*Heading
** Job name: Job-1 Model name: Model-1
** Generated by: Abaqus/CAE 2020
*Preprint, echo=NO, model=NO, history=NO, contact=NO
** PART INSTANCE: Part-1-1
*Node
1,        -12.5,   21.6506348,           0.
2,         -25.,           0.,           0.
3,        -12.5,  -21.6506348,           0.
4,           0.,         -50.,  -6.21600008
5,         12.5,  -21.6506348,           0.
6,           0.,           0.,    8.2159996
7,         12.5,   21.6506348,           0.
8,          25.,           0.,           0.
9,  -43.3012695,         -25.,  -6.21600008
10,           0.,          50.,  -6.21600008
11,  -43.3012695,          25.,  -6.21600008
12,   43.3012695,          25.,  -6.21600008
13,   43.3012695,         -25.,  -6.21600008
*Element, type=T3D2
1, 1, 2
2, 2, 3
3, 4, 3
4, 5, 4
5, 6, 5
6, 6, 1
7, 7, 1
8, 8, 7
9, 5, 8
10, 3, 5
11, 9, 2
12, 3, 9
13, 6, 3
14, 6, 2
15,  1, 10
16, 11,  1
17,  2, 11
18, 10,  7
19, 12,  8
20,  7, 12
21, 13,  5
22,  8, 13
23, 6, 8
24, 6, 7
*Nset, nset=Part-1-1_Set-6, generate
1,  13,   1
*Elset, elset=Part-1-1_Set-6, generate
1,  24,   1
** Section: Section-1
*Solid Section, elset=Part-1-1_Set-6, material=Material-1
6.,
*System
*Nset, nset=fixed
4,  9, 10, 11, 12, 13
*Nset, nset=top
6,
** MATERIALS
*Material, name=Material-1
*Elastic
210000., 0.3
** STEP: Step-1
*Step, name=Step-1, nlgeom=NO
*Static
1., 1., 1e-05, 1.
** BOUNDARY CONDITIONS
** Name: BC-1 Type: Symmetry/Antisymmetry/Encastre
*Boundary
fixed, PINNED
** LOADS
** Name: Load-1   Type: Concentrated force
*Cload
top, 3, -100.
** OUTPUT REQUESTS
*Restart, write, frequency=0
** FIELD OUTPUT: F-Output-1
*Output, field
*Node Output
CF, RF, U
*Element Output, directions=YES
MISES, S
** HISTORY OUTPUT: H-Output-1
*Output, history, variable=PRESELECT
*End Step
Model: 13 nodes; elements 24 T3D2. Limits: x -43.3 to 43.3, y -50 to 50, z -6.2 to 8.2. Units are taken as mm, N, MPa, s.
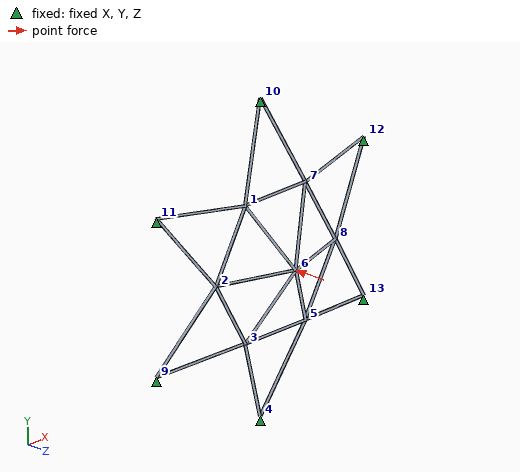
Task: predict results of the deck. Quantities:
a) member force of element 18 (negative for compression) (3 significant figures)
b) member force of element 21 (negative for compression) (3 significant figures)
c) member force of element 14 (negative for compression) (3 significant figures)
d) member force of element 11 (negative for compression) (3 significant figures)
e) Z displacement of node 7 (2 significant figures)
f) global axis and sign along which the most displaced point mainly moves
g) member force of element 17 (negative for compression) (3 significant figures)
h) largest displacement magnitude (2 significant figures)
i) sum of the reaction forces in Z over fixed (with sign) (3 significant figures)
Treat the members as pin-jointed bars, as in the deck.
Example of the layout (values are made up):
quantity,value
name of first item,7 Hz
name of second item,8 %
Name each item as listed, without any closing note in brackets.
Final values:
quantity,value
member force of element 18 (negative for compression),-42.4 N
member force of element 21 (negative for compression),-42.4 N
member force of element 14 (negative for compression),-53.4 N
member force of element 11 (negative for compression),-42.4 N
Z displacement of node 7,-0.0053 mm
global axis and sign along which the most displaced point mainly moves,-Z
member force of element 17 (negative for compression),-42.4 N
largest displacement magnitude,0.0090 mm
sum of the reaction forces in Z over fixed (with sign),100 N
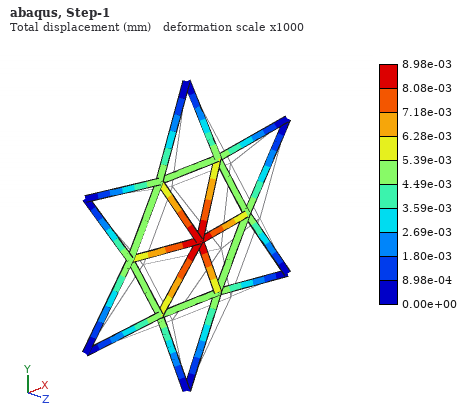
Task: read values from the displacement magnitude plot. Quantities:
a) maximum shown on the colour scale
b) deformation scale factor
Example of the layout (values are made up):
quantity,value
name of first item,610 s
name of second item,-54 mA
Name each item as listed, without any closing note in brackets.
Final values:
quantity,value
maximum shown on the colour scale,8.98e-03 mm
deformation scale factor,1000
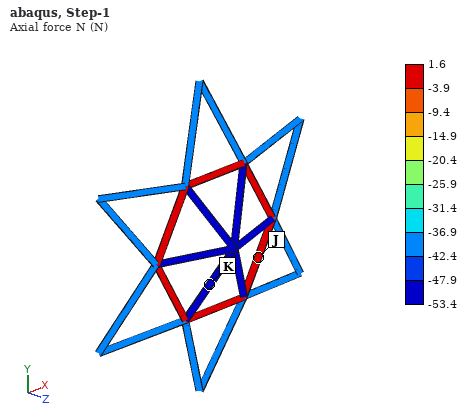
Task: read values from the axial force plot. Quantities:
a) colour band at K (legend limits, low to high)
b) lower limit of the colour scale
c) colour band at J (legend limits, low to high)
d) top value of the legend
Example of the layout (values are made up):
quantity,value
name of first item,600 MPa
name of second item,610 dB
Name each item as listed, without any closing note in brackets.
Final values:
quantity,value
colour band at K,-53.4 to -47.9 N
lower limit of the colour scale,-53.4 N
colour band at J,-3.9 to 1.6 N
top value of the legend,1.6 N
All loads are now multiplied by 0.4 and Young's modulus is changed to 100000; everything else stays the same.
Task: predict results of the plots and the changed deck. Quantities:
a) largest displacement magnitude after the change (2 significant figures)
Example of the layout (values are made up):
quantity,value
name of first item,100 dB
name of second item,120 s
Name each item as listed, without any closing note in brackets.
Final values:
quantity,value
largest displacement magnitude after the change,0.0075 mm
